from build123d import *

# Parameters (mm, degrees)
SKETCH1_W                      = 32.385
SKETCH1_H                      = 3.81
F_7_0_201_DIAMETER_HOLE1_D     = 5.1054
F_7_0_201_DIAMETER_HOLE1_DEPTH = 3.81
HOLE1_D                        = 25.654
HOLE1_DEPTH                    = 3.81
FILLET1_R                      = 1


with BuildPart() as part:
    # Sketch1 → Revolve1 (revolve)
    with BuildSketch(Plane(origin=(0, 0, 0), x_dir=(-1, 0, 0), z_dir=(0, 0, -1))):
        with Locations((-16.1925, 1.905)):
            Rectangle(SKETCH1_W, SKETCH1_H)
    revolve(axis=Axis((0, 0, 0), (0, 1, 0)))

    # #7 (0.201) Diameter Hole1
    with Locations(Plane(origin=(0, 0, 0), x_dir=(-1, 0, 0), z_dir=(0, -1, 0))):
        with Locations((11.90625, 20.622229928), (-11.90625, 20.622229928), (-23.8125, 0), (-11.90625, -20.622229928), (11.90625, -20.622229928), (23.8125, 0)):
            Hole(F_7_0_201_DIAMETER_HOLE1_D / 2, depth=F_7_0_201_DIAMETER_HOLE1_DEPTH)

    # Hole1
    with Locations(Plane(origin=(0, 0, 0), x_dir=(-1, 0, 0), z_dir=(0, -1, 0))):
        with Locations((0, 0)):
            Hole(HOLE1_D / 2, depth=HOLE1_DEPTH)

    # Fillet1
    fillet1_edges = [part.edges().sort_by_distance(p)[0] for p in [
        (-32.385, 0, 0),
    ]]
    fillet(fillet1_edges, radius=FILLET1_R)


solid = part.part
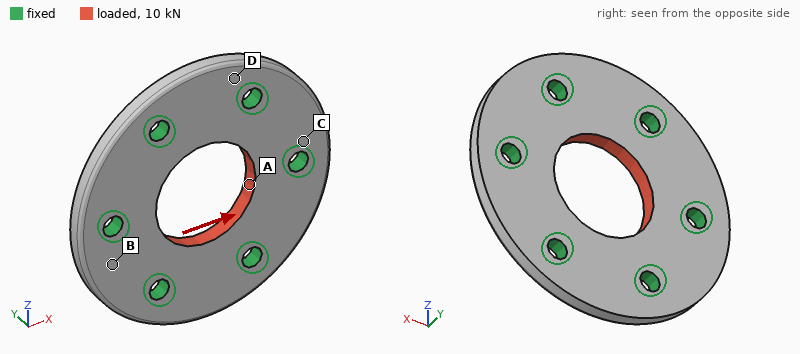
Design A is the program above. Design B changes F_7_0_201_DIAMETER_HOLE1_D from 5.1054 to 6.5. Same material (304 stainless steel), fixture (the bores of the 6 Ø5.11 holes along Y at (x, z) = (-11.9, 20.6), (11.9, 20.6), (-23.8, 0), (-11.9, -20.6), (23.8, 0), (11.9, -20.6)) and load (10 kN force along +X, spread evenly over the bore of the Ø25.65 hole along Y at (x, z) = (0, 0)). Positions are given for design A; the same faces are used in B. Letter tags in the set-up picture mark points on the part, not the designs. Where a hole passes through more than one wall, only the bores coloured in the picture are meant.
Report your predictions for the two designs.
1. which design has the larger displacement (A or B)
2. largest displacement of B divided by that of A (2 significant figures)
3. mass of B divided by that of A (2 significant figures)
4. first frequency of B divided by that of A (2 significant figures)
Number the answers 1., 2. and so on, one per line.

1. A
2. 0.91
3. 0.97
4. 1.2
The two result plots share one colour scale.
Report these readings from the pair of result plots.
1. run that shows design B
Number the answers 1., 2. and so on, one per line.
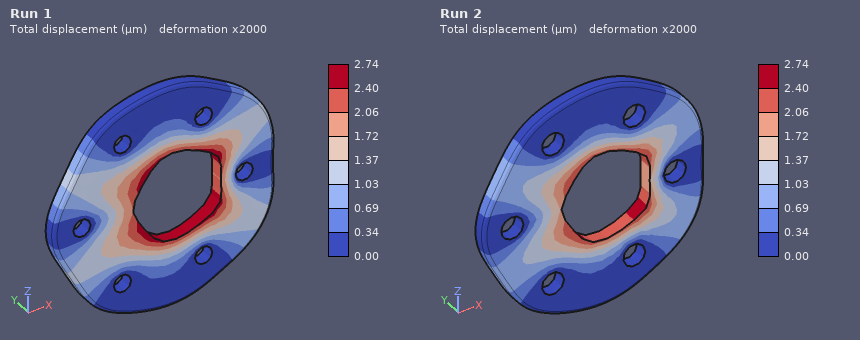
1. Run 2
